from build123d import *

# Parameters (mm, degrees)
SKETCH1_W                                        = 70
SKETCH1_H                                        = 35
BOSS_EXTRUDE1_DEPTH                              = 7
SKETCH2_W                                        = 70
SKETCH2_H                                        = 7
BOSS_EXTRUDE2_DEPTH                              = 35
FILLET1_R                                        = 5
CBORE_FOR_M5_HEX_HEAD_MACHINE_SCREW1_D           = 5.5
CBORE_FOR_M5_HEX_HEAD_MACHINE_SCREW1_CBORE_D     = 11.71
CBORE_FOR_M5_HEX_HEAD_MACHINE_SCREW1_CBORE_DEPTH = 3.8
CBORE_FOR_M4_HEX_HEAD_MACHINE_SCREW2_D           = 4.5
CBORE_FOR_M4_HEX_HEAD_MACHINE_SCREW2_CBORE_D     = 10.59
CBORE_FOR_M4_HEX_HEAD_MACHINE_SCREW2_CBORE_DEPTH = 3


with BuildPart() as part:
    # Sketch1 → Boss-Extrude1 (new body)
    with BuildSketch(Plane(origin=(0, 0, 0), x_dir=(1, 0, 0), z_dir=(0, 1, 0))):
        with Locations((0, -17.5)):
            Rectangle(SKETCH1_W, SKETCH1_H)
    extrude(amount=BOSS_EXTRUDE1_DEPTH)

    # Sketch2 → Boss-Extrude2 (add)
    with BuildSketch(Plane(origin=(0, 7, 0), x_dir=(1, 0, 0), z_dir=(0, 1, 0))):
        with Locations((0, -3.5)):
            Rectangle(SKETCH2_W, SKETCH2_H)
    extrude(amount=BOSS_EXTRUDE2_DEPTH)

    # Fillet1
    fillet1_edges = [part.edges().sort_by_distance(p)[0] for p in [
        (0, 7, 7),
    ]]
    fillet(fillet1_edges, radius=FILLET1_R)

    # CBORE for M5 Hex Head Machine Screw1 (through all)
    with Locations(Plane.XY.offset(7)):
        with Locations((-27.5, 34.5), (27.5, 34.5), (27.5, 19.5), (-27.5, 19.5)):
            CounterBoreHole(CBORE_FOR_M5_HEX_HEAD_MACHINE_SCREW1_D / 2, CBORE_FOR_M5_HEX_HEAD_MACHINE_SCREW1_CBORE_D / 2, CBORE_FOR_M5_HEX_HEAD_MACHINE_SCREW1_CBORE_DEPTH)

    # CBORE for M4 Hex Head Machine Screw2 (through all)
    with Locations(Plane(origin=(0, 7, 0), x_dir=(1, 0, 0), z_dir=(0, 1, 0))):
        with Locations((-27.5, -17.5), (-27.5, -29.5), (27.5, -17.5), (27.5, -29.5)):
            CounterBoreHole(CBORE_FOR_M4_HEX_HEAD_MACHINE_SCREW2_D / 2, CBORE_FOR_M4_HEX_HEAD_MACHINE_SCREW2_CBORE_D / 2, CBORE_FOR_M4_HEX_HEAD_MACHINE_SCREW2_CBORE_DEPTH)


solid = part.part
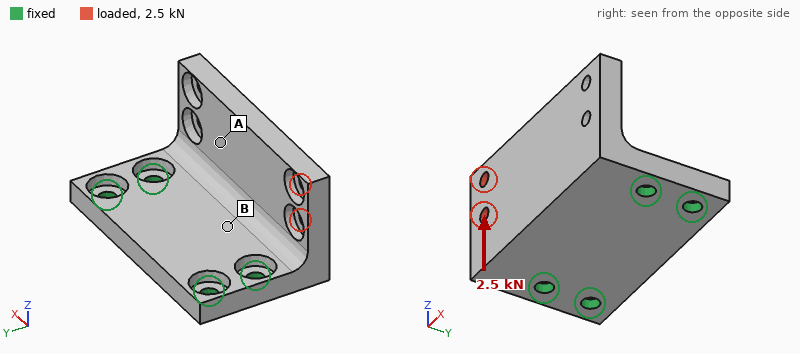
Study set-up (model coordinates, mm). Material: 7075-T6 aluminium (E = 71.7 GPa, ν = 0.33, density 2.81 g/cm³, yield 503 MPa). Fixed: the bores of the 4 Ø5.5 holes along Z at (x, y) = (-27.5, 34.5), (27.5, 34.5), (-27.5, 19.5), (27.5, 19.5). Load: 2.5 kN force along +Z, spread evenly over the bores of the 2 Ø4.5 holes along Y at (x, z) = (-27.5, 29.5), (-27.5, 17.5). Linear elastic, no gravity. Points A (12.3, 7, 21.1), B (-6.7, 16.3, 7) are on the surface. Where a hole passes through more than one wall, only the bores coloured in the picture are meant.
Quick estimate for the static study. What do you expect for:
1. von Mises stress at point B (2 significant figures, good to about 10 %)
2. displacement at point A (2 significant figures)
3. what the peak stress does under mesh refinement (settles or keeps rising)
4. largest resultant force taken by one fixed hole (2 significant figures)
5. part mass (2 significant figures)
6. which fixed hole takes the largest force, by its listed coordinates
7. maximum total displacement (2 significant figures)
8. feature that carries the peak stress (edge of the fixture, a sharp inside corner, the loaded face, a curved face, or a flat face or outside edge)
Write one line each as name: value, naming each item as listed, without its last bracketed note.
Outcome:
von Mises stress at point B: 52 MPa
displacement at point A: 0.092 mm
what the peak stress does under mesh refinement: keeps rising
largest resultant force taken by one fixed hole: 3.8 kN
part mass: 88 g
which fixed hole takes the largest force, by its listed coordinates: (-27.5, 19.5)
maximum total displacement: 0.30 mm
feature that carries the peak stress: edge of the fixture
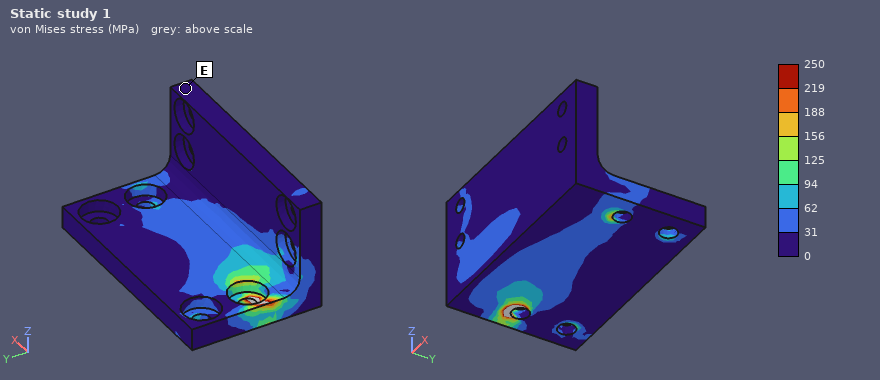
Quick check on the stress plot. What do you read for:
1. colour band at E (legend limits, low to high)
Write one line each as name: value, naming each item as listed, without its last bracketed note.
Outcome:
colour band at E: 0 to 31 MPa
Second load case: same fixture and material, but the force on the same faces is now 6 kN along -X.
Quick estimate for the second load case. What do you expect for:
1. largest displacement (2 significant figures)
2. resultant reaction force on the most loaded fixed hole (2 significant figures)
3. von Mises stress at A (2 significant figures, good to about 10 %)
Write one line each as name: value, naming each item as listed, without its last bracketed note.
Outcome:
largest displacement: 0.14 mm
resultant reaction force on the most loaded fixed hole: 4.0 kN
von Mises stress at A: 40 MPa
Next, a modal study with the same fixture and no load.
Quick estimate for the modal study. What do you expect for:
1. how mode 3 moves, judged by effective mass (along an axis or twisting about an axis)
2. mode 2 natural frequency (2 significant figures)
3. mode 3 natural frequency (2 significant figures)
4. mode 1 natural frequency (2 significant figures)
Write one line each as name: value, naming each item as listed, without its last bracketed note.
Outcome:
how mode 3 moves, judged by effective mass: along Z
mode 2 natural frequency: 5200 Hz
mode 3 natural frequency: 7700 Hz
mode 1 natural frequency: 2700 Hz
